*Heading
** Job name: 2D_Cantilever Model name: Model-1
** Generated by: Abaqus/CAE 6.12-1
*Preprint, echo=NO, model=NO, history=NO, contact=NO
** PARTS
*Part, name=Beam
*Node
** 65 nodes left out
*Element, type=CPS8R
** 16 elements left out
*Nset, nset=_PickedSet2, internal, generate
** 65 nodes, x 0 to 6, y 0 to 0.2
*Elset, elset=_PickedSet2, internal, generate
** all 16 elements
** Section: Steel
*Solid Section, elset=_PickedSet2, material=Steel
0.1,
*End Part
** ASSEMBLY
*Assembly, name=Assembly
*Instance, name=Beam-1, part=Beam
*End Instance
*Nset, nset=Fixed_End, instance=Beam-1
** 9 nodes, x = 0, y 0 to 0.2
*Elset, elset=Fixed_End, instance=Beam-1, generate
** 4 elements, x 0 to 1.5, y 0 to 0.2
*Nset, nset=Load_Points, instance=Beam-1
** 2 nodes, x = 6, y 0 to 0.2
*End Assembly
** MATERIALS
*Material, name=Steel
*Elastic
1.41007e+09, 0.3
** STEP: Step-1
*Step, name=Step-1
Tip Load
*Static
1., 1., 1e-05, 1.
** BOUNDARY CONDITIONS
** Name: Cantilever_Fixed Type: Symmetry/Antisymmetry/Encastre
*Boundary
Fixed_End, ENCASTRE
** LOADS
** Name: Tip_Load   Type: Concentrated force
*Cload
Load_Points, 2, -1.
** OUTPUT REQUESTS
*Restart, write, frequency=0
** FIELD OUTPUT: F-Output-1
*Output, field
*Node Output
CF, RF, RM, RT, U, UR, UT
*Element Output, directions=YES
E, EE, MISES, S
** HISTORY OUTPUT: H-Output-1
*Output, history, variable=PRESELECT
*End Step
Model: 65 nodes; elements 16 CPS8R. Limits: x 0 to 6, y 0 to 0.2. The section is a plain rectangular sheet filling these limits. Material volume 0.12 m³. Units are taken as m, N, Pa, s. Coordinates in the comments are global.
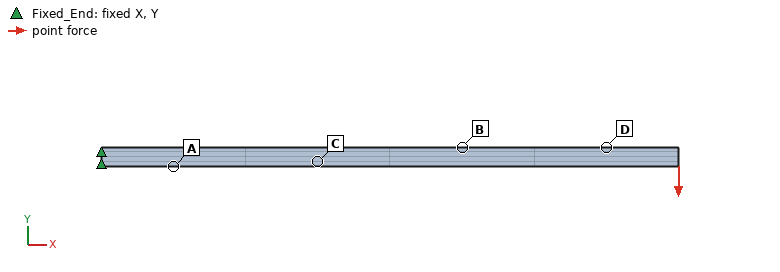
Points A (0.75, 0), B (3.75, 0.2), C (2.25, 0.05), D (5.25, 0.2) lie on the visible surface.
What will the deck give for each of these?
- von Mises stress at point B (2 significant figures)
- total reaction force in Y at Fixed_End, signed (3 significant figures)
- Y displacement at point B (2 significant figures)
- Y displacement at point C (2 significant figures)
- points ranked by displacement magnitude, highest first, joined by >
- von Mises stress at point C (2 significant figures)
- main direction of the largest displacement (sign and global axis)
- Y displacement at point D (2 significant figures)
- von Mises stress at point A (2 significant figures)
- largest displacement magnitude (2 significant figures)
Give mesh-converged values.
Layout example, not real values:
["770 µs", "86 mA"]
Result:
["6600 Pa", "2.00 N", "-7.1e-04 m", "-2.8e-04 m", "D > B > C > A", "5600 Pa", "-Y", "-0.0012 m", "16000 Pa", "0.0015 m"]
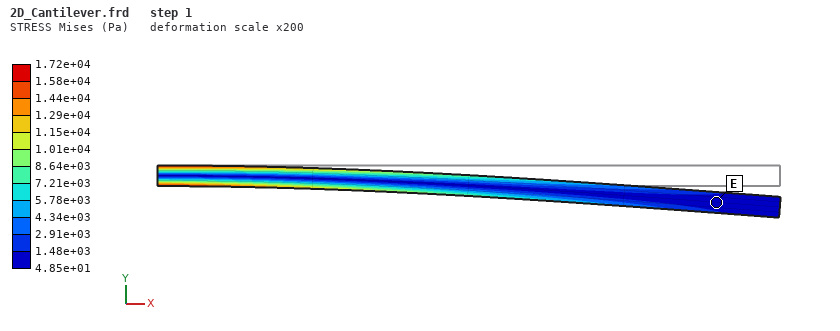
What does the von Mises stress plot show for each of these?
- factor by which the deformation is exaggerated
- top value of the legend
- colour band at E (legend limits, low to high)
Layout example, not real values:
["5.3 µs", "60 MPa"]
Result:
["200", "1.72e+04 Pa", "4.85e+01 to 1.48e+03 Pa"]
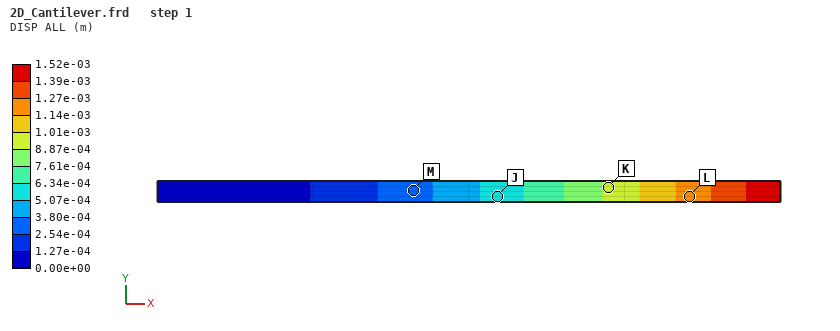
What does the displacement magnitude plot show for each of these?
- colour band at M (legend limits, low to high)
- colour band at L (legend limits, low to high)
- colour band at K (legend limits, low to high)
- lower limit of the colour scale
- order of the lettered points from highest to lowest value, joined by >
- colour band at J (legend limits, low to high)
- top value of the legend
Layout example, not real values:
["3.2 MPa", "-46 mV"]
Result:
["2.54e-04 to 3.80e-04 m", "1.14e-03 to 1.27e-03 m", "8.87e-04 to 1.01e-03 m", "0.00e+00 m", "L > K > J > M", "5.07e-04 to 6.34e-04 m", "1.52e-03 m"]
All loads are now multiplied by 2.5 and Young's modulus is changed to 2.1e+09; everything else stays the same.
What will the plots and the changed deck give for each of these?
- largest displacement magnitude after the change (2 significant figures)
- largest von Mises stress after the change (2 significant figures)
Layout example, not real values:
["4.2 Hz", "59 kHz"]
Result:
["0.0026 m", "43000 Pa"]
